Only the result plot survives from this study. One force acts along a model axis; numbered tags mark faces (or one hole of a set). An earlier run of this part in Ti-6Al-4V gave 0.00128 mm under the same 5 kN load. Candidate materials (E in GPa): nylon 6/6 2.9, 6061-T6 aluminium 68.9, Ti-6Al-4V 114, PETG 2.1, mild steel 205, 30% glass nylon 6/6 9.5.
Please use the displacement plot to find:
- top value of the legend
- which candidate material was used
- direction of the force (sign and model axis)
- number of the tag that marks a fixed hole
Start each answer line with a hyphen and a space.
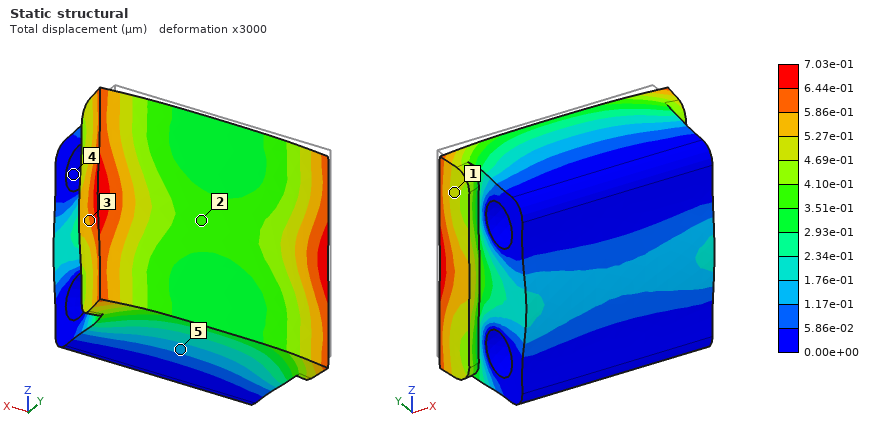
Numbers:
- 7.03e-01 µm
- mild steel
- -Y
- 4
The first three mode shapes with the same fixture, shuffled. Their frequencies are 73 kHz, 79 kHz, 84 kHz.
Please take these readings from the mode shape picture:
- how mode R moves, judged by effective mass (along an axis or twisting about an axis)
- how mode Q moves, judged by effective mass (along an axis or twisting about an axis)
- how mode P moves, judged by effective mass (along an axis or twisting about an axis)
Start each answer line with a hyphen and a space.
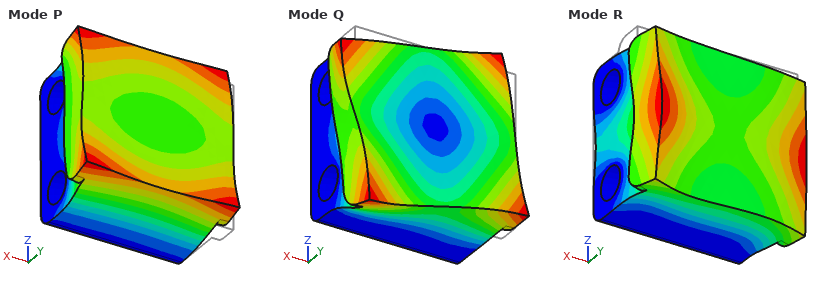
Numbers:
- along X
- twisting about Y
- along Z
